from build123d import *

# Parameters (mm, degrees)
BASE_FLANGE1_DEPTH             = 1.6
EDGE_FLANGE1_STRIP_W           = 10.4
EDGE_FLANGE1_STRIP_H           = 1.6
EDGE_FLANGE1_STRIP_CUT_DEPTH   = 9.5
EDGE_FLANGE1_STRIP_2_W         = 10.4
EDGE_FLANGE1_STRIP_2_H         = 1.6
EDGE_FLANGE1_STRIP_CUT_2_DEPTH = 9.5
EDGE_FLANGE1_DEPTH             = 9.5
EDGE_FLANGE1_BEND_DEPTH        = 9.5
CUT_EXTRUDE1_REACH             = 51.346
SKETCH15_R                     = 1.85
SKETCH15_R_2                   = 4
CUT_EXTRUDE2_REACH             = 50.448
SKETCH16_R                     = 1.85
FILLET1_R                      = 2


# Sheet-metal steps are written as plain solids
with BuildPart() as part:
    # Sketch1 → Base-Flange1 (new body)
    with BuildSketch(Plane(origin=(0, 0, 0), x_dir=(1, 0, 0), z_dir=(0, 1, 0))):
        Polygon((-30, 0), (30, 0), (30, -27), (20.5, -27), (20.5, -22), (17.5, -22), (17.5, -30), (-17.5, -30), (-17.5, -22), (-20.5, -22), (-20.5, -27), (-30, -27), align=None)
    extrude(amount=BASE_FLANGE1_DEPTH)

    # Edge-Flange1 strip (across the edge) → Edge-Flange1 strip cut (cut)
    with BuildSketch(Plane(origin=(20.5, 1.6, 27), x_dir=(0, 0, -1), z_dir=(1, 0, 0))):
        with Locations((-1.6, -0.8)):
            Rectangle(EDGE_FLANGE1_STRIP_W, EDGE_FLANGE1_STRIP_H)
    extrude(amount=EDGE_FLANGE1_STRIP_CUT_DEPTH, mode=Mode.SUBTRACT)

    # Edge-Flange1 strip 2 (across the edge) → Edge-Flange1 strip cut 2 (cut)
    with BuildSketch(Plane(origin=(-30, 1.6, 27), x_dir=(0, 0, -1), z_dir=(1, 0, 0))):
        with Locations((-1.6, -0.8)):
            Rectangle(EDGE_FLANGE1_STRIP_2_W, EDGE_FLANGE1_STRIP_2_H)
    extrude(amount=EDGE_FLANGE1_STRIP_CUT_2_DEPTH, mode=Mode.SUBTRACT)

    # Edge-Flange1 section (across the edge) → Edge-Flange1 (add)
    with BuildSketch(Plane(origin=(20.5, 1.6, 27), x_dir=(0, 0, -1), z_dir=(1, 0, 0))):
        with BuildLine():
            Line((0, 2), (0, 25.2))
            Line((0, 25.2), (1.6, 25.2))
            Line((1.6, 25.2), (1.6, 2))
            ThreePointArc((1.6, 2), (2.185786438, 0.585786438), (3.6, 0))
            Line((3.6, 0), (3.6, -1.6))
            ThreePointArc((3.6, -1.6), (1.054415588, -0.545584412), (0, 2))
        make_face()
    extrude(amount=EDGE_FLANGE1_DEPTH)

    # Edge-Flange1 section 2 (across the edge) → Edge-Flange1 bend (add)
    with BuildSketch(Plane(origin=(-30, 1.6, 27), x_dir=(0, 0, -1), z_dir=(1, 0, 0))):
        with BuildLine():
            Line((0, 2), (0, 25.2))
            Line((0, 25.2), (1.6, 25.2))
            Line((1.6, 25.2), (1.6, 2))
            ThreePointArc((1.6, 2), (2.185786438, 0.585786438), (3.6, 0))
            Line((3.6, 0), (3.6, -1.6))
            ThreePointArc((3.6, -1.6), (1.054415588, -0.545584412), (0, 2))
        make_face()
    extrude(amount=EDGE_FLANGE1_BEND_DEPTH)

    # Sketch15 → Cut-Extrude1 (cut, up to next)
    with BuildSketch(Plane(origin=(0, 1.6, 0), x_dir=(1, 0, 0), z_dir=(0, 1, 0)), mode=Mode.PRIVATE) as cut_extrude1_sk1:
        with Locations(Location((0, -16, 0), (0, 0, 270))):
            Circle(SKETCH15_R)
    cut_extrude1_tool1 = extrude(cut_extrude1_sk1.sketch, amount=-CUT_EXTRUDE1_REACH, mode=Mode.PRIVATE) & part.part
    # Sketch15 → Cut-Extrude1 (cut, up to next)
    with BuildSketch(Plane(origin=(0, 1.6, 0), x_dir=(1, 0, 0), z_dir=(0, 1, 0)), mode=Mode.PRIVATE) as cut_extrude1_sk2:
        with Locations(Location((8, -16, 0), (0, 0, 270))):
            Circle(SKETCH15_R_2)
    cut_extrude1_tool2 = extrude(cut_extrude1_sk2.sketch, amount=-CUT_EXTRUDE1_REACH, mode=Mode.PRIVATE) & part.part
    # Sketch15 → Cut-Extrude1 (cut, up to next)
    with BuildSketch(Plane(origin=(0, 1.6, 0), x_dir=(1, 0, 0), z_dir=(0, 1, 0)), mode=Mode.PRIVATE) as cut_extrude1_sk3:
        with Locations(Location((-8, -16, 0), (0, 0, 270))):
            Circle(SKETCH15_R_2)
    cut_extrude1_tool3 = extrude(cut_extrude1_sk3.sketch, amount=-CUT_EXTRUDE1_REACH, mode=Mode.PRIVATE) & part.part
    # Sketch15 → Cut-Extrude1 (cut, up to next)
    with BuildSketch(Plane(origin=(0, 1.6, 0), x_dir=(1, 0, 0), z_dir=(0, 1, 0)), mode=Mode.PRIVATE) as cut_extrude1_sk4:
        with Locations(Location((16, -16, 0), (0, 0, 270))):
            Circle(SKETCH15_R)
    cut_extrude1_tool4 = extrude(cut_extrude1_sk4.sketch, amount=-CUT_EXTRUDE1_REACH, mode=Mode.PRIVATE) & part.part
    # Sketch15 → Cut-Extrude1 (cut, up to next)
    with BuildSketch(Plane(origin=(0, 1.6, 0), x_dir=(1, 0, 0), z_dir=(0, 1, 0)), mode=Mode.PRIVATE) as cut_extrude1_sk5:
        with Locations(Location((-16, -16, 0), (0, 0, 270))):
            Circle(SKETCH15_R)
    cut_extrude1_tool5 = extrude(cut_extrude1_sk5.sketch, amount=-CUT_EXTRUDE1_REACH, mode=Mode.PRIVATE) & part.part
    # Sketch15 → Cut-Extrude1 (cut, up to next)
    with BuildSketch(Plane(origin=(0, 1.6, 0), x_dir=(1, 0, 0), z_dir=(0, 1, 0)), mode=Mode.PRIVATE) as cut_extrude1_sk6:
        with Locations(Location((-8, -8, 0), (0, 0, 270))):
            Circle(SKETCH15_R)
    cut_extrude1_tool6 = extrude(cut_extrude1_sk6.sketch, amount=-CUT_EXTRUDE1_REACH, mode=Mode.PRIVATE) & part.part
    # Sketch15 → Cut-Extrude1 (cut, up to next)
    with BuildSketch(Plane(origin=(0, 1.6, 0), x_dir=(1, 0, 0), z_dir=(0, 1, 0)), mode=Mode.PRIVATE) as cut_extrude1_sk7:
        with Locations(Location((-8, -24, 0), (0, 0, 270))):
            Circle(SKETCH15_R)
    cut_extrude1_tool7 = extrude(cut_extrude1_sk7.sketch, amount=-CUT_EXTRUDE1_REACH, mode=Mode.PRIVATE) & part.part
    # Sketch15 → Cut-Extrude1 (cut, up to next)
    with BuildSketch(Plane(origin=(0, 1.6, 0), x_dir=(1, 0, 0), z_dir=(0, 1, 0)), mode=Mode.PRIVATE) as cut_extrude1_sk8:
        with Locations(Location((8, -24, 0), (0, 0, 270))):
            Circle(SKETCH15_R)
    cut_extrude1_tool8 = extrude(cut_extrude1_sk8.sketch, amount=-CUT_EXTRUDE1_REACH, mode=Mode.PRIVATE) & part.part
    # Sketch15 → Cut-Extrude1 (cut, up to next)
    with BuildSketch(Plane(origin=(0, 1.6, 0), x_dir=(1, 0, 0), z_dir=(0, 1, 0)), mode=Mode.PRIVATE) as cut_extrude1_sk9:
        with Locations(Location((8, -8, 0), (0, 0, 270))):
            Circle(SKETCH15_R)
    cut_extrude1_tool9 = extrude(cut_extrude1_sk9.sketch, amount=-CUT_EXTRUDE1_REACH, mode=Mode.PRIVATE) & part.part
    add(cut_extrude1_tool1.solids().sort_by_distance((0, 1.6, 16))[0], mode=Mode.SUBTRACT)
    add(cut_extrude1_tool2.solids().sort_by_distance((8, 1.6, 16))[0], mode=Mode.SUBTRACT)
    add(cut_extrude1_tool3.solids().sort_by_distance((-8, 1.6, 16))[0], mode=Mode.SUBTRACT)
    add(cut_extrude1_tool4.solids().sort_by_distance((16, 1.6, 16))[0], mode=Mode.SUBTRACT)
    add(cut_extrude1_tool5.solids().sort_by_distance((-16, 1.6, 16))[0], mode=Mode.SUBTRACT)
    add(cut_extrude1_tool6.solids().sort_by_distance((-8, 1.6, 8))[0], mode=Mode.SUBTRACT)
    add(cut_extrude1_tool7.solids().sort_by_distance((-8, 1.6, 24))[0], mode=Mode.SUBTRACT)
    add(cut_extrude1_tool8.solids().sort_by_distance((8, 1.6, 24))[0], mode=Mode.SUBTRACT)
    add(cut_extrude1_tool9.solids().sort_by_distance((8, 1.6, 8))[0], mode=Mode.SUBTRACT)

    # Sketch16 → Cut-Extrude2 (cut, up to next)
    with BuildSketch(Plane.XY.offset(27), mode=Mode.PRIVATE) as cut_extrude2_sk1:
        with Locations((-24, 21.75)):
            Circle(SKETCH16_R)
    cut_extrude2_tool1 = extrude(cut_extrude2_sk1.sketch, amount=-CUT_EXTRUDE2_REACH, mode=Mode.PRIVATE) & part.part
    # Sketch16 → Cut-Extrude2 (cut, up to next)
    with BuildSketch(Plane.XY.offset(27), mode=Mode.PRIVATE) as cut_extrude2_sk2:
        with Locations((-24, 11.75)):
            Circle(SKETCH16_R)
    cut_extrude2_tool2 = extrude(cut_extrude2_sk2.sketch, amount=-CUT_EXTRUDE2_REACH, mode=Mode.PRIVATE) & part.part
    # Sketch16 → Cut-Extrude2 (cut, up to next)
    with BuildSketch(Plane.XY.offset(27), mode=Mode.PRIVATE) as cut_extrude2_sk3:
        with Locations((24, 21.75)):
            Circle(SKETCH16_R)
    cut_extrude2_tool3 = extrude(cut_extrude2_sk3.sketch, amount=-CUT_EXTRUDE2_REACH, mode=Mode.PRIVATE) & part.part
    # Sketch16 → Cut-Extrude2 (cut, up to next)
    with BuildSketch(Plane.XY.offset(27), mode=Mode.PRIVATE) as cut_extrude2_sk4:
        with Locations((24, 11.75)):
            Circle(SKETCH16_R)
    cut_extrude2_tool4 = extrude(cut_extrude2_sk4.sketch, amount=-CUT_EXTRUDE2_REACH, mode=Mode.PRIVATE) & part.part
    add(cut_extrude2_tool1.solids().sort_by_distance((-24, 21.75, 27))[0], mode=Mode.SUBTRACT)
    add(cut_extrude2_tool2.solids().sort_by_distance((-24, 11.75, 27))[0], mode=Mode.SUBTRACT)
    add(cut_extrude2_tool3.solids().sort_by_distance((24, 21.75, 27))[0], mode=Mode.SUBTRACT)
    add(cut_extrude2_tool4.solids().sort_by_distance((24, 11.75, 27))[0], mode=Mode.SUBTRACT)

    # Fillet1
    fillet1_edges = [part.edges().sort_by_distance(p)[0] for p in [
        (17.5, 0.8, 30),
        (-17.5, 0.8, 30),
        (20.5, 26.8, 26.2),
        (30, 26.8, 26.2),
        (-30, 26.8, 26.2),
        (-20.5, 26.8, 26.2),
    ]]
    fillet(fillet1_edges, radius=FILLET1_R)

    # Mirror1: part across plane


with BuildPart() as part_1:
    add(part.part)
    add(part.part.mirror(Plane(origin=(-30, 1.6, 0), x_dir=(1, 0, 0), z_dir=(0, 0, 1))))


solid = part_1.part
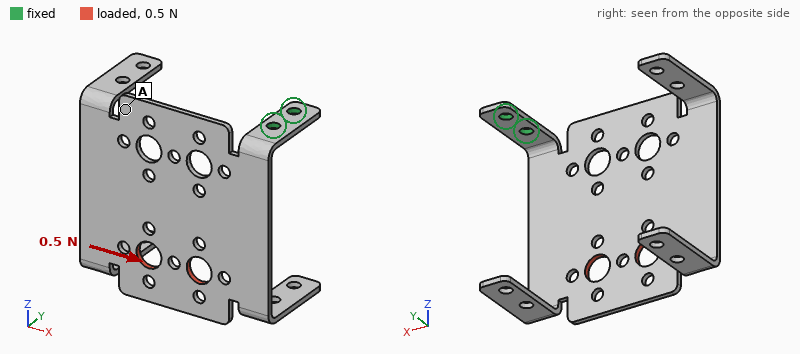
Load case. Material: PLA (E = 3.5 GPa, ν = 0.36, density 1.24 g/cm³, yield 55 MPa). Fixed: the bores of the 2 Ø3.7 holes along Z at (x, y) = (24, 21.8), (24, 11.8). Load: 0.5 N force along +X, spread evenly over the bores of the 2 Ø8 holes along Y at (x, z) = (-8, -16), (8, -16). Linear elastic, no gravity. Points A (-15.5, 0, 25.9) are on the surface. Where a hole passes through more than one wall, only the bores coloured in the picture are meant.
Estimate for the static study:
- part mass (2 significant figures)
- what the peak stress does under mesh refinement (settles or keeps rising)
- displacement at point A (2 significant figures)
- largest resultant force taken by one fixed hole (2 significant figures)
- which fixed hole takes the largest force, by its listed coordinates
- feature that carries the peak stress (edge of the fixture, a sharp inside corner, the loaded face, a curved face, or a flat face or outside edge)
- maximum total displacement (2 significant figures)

7.6 g
keeps rising
0.45 mm
0.76 N
(24, 11.8)
edge of the fixture
0.89 mm
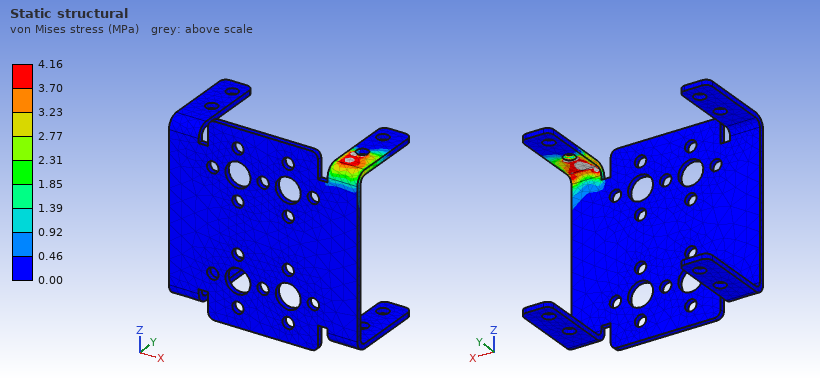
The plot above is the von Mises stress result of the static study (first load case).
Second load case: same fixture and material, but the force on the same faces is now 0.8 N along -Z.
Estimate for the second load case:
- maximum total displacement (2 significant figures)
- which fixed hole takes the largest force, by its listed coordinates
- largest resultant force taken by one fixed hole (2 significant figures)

0.86 mm
(24, 11.8)
0.61 N
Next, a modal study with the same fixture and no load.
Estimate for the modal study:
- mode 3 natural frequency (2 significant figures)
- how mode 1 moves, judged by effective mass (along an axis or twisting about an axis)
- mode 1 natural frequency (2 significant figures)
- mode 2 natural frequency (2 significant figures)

82 Hz
along Y
39 Hz
55 Hz
